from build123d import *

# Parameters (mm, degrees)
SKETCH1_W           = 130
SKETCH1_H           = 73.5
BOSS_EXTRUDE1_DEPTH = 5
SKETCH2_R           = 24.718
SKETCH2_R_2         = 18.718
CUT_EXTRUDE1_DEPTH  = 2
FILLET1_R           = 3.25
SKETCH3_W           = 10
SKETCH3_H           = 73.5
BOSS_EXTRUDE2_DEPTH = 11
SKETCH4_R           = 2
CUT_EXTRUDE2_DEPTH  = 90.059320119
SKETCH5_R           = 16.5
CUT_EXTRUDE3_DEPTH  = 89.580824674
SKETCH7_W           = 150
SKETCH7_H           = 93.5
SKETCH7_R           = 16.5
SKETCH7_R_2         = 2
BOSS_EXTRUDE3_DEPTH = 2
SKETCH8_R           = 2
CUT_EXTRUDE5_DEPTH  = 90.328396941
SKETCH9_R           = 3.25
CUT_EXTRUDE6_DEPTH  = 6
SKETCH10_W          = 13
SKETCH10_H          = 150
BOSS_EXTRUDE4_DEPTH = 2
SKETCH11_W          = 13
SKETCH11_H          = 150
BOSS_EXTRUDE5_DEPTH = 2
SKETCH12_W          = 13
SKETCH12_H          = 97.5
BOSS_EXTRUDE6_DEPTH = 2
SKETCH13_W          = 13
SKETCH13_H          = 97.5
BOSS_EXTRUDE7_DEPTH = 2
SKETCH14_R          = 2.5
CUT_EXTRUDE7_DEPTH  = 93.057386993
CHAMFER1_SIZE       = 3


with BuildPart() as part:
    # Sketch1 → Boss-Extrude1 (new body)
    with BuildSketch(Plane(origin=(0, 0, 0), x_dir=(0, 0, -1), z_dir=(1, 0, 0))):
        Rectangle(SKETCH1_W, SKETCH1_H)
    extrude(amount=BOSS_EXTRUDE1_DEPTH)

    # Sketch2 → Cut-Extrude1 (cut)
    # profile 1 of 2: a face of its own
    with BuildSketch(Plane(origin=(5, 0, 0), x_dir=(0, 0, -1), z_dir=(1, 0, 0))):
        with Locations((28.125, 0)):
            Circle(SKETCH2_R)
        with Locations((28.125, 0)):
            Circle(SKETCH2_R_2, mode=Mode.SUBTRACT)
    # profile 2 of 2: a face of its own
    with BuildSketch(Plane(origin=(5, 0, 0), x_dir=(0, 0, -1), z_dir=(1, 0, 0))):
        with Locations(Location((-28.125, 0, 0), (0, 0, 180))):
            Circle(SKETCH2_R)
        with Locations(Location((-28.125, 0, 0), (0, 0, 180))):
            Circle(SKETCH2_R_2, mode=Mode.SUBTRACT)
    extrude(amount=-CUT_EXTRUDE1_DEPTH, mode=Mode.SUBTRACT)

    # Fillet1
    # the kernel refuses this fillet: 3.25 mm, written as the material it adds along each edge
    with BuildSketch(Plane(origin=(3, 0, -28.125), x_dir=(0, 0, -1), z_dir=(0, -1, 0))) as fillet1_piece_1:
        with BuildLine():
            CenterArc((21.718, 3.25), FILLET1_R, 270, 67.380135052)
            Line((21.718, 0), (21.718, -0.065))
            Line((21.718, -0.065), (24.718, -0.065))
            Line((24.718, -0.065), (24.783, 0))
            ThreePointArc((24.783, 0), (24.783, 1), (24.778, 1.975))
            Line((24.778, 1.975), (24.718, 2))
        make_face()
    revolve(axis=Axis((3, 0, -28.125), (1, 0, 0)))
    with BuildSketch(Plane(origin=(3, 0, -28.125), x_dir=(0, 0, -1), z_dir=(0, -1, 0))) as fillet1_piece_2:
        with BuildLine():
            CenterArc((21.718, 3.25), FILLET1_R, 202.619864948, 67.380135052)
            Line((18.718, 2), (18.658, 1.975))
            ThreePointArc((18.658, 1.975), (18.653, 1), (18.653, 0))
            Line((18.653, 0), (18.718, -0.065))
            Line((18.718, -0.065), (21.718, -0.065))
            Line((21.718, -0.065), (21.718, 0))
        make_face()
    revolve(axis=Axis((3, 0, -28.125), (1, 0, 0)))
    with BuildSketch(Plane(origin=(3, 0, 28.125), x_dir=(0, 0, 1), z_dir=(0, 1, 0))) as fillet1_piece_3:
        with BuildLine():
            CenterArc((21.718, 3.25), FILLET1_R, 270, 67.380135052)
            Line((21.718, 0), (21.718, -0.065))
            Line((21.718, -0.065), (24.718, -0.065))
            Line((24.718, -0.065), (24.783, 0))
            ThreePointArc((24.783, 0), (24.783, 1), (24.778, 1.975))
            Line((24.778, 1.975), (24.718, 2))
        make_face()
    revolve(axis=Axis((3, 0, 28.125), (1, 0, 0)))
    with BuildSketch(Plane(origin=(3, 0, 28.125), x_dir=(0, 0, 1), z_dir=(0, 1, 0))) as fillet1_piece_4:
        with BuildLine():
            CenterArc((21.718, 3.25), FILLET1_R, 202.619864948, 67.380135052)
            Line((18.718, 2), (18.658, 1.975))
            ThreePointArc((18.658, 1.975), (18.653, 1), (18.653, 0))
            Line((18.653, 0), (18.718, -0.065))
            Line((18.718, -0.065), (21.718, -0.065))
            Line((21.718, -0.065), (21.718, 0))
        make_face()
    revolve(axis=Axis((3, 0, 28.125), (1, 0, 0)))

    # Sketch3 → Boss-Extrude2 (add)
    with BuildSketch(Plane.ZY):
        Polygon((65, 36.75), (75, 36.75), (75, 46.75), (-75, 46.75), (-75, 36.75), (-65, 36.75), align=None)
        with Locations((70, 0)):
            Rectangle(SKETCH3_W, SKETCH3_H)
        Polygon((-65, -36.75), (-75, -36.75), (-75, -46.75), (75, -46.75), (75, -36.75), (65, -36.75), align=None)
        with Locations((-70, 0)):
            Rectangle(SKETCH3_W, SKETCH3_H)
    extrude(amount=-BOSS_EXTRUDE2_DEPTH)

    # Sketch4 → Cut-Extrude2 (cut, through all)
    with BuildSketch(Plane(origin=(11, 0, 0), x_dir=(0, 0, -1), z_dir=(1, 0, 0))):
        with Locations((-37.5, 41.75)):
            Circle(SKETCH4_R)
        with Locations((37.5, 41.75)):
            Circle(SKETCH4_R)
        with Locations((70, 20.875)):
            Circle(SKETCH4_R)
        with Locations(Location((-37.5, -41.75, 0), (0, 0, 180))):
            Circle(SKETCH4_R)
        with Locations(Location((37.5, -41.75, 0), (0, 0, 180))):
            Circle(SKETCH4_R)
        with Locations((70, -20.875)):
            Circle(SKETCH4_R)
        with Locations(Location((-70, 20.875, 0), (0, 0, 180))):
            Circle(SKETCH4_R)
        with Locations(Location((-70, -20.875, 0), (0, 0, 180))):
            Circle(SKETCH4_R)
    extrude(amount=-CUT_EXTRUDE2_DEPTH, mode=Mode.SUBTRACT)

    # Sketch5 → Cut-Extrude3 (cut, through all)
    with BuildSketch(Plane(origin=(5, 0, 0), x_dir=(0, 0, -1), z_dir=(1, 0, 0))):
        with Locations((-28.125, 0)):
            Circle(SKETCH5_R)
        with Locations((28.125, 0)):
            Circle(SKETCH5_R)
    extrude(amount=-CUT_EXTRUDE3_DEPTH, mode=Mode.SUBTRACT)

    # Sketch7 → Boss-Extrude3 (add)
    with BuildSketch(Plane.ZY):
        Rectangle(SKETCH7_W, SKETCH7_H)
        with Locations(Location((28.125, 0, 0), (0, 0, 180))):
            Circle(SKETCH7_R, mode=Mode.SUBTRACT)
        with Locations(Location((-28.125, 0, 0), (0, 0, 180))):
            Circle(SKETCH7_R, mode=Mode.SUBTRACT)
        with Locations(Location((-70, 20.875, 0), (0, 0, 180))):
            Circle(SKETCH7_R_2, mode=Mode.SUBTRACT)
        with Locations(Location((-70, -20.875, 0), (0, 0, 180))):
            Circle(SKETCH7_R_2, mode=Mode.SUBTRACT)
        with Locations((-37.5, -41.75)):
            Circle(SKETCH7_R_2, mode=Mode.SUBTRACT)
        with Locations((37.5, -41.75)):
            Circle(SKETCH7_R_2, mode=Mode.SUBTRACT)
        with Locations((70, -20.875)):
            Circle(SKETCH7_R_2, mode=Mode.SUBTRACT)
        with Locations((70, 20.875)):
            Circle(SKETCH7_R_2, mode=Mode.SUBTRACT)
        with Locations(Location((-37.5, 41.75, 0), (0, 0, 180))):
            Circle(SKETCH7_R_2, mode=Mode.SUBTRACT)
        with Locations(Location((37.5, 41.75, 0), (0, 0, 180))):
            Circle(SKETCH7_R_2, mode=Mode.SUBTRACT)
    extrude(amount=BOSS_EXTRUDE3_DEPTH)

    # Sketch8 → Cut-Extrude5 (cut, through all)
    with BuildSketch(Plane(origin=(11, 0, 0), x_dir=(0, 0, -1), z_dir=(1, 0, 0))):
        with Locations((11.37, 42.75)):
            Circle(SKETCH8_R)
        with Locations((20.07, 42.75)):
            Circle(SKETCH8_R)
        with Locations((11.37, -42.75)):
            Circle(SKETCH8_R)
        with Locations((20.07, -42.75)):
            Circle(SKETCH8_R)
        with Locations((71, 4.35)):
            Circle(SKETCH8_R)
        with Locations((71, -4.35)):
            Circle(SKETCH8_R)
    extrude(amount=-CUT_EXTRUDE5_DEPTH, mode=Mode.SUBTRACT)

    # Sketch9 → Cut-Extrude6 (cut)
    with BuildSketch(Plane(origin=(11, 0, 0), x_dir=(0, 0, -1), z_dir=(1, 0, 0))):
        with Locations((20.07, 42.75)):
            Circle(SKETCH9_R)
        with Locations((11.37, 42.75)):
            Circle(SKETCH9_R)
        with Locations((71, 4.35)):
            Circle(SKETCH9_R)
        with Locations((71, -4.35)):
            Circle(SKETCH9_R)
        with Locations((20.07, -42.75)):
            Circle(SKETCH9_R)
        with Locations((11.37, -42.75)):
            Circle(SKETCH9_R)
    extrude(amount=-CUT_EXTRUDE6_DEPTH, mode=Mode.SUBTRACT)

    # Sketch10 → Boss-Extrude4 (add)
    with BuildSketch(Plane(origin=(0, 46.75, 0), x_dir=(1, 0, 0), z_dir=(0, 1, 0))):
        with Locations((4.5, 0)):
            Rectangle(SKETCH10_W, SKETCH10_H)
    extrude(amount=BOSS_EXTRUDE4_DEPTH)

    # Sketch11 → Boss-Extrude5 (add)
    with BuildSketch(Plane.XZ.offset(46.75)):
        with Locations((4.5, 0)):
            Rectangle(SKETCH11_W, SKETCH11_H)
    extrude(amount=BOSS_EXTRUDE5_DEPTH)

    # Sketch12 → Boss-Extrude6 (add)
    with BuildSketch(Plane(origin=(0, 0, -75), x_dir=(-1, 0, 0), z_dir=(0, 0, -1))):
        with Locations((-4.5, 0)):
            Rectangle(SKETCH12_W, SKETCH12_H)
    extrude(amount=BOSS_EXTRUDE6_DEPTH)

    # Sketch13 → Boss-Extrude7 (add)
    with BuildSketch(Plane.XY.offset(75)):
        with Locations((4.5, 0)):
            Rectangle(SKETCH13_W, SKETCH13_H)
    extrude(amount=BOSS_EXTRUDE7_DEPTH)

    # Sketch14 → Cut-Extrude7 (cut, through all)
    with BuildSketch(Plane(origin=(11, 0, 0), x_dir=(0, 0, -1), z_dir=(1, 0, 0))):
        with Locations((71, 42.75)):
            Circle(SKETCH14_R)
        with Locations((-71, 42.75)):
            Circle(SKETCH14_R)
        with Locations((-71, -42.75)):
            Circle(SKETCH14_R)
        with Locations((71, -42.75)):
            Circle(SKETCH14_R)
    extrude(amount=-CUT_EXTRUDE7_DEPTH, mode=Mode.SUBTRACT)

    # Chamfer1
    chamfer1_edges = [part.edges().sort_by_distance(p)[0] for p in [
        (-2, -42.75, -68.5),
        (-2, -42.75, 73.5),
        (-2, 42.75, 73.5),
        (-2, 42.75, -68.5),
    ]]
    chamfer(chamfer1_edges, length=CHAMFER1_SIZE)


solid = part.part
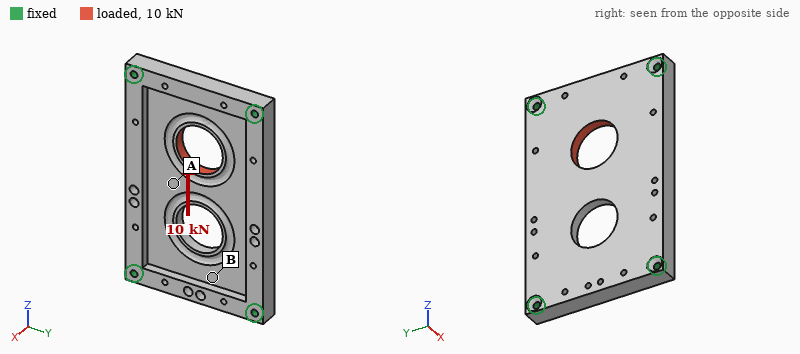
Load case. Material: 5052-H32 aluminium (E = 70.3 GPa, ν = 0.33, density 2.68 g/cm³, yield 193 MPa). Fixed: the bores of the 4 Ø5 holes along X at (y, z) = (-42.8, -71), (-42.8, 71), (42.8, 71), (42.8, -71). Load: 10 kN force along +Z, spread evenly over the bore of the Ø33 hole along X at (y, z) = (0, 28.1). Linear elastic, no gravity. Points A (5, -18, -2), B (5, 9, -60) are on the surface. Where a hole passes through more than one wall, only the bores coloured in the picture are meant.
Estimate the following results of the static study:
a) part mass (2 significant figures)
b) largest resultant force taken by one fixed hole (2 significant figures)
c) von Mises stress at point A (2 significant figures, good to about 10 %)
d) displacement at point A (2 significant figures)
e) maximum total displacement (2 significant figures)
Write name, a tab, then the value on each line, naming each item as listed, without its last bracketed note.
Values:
part mass	320 g
largest resultant force taken by one fixed hole	3.3 kN
von Mises stress at point A	14 MPa
displacement at point A	12 µm
maximum total displacement	24 µm
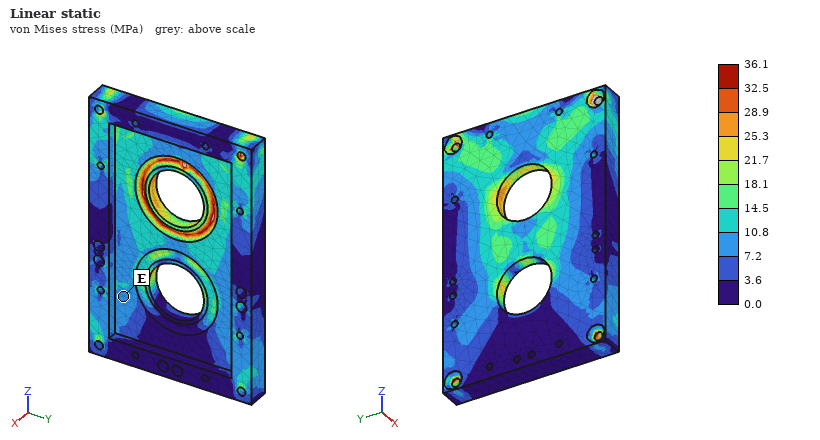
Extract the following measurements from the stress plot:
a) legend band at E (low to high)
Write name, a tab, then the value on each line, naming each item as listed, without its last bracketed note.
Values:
legend band at E	7.2 to 10.8 MPa
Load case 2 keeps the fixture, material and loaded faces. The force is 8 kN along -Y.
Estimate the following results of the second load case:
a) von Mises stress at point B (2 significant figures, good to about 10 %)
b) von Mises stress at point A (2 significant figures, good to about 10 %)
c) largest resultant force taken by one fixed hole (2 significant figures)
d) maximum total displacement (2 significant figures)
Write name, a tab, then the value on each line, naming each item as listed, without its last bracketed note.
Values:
von Mises stress at point B	9.4 MPa
von Mises stress at point A	8.4 MPa
largest resultant force taken by one fixed hole	3.3 kN
maximum total displacement	29 µm
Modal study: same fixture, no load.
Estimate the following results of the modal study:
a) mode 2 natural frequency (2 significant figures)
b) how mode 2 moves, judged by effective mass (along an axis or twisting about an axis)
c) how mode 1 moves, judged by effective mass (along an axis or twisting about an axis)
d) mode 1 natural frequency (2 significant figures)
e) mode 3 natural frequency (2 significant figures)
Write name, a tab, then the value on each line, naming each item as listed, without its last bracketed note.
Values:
mode 2 natural frequency	3100 Hz
how mode 2 moves, judged by effective mass	twisting about Z
how mode 1 moves, judged by effective mass	along X
mode 1 natural frequency	2300 Hz
mode 3 natural frequency	5000 Hz
